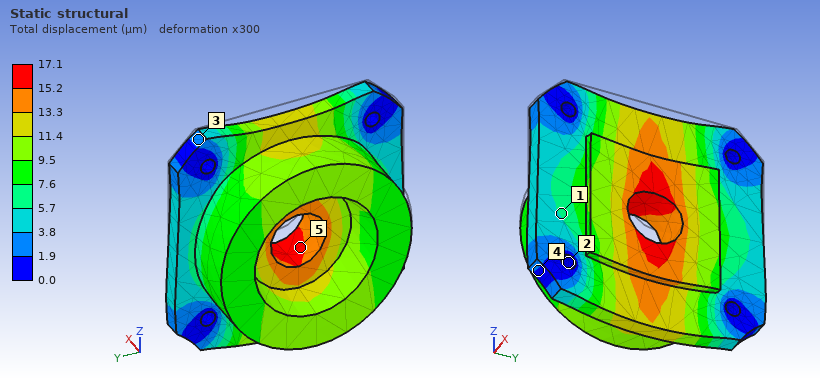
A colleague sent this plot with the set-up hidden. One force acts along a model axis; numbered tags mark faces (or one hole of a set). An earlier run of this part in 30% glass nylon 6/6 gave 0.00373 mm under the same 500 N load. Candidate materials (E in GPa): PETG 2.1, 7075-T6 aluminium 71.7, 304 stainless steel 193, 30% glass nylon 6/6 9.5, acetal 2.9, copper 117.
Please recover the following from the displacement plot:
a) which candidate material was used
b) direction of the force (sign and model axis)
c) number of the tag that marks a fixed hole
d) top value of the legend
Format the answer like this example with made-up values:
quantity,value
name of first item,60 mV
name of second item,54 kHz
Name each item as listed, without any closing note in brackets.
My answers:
quantity,value
which candidate material was used,PETG
direction of the force,-Z
number of the tag that marks a fixed hole,2
top value of the legend,17.1 µm
